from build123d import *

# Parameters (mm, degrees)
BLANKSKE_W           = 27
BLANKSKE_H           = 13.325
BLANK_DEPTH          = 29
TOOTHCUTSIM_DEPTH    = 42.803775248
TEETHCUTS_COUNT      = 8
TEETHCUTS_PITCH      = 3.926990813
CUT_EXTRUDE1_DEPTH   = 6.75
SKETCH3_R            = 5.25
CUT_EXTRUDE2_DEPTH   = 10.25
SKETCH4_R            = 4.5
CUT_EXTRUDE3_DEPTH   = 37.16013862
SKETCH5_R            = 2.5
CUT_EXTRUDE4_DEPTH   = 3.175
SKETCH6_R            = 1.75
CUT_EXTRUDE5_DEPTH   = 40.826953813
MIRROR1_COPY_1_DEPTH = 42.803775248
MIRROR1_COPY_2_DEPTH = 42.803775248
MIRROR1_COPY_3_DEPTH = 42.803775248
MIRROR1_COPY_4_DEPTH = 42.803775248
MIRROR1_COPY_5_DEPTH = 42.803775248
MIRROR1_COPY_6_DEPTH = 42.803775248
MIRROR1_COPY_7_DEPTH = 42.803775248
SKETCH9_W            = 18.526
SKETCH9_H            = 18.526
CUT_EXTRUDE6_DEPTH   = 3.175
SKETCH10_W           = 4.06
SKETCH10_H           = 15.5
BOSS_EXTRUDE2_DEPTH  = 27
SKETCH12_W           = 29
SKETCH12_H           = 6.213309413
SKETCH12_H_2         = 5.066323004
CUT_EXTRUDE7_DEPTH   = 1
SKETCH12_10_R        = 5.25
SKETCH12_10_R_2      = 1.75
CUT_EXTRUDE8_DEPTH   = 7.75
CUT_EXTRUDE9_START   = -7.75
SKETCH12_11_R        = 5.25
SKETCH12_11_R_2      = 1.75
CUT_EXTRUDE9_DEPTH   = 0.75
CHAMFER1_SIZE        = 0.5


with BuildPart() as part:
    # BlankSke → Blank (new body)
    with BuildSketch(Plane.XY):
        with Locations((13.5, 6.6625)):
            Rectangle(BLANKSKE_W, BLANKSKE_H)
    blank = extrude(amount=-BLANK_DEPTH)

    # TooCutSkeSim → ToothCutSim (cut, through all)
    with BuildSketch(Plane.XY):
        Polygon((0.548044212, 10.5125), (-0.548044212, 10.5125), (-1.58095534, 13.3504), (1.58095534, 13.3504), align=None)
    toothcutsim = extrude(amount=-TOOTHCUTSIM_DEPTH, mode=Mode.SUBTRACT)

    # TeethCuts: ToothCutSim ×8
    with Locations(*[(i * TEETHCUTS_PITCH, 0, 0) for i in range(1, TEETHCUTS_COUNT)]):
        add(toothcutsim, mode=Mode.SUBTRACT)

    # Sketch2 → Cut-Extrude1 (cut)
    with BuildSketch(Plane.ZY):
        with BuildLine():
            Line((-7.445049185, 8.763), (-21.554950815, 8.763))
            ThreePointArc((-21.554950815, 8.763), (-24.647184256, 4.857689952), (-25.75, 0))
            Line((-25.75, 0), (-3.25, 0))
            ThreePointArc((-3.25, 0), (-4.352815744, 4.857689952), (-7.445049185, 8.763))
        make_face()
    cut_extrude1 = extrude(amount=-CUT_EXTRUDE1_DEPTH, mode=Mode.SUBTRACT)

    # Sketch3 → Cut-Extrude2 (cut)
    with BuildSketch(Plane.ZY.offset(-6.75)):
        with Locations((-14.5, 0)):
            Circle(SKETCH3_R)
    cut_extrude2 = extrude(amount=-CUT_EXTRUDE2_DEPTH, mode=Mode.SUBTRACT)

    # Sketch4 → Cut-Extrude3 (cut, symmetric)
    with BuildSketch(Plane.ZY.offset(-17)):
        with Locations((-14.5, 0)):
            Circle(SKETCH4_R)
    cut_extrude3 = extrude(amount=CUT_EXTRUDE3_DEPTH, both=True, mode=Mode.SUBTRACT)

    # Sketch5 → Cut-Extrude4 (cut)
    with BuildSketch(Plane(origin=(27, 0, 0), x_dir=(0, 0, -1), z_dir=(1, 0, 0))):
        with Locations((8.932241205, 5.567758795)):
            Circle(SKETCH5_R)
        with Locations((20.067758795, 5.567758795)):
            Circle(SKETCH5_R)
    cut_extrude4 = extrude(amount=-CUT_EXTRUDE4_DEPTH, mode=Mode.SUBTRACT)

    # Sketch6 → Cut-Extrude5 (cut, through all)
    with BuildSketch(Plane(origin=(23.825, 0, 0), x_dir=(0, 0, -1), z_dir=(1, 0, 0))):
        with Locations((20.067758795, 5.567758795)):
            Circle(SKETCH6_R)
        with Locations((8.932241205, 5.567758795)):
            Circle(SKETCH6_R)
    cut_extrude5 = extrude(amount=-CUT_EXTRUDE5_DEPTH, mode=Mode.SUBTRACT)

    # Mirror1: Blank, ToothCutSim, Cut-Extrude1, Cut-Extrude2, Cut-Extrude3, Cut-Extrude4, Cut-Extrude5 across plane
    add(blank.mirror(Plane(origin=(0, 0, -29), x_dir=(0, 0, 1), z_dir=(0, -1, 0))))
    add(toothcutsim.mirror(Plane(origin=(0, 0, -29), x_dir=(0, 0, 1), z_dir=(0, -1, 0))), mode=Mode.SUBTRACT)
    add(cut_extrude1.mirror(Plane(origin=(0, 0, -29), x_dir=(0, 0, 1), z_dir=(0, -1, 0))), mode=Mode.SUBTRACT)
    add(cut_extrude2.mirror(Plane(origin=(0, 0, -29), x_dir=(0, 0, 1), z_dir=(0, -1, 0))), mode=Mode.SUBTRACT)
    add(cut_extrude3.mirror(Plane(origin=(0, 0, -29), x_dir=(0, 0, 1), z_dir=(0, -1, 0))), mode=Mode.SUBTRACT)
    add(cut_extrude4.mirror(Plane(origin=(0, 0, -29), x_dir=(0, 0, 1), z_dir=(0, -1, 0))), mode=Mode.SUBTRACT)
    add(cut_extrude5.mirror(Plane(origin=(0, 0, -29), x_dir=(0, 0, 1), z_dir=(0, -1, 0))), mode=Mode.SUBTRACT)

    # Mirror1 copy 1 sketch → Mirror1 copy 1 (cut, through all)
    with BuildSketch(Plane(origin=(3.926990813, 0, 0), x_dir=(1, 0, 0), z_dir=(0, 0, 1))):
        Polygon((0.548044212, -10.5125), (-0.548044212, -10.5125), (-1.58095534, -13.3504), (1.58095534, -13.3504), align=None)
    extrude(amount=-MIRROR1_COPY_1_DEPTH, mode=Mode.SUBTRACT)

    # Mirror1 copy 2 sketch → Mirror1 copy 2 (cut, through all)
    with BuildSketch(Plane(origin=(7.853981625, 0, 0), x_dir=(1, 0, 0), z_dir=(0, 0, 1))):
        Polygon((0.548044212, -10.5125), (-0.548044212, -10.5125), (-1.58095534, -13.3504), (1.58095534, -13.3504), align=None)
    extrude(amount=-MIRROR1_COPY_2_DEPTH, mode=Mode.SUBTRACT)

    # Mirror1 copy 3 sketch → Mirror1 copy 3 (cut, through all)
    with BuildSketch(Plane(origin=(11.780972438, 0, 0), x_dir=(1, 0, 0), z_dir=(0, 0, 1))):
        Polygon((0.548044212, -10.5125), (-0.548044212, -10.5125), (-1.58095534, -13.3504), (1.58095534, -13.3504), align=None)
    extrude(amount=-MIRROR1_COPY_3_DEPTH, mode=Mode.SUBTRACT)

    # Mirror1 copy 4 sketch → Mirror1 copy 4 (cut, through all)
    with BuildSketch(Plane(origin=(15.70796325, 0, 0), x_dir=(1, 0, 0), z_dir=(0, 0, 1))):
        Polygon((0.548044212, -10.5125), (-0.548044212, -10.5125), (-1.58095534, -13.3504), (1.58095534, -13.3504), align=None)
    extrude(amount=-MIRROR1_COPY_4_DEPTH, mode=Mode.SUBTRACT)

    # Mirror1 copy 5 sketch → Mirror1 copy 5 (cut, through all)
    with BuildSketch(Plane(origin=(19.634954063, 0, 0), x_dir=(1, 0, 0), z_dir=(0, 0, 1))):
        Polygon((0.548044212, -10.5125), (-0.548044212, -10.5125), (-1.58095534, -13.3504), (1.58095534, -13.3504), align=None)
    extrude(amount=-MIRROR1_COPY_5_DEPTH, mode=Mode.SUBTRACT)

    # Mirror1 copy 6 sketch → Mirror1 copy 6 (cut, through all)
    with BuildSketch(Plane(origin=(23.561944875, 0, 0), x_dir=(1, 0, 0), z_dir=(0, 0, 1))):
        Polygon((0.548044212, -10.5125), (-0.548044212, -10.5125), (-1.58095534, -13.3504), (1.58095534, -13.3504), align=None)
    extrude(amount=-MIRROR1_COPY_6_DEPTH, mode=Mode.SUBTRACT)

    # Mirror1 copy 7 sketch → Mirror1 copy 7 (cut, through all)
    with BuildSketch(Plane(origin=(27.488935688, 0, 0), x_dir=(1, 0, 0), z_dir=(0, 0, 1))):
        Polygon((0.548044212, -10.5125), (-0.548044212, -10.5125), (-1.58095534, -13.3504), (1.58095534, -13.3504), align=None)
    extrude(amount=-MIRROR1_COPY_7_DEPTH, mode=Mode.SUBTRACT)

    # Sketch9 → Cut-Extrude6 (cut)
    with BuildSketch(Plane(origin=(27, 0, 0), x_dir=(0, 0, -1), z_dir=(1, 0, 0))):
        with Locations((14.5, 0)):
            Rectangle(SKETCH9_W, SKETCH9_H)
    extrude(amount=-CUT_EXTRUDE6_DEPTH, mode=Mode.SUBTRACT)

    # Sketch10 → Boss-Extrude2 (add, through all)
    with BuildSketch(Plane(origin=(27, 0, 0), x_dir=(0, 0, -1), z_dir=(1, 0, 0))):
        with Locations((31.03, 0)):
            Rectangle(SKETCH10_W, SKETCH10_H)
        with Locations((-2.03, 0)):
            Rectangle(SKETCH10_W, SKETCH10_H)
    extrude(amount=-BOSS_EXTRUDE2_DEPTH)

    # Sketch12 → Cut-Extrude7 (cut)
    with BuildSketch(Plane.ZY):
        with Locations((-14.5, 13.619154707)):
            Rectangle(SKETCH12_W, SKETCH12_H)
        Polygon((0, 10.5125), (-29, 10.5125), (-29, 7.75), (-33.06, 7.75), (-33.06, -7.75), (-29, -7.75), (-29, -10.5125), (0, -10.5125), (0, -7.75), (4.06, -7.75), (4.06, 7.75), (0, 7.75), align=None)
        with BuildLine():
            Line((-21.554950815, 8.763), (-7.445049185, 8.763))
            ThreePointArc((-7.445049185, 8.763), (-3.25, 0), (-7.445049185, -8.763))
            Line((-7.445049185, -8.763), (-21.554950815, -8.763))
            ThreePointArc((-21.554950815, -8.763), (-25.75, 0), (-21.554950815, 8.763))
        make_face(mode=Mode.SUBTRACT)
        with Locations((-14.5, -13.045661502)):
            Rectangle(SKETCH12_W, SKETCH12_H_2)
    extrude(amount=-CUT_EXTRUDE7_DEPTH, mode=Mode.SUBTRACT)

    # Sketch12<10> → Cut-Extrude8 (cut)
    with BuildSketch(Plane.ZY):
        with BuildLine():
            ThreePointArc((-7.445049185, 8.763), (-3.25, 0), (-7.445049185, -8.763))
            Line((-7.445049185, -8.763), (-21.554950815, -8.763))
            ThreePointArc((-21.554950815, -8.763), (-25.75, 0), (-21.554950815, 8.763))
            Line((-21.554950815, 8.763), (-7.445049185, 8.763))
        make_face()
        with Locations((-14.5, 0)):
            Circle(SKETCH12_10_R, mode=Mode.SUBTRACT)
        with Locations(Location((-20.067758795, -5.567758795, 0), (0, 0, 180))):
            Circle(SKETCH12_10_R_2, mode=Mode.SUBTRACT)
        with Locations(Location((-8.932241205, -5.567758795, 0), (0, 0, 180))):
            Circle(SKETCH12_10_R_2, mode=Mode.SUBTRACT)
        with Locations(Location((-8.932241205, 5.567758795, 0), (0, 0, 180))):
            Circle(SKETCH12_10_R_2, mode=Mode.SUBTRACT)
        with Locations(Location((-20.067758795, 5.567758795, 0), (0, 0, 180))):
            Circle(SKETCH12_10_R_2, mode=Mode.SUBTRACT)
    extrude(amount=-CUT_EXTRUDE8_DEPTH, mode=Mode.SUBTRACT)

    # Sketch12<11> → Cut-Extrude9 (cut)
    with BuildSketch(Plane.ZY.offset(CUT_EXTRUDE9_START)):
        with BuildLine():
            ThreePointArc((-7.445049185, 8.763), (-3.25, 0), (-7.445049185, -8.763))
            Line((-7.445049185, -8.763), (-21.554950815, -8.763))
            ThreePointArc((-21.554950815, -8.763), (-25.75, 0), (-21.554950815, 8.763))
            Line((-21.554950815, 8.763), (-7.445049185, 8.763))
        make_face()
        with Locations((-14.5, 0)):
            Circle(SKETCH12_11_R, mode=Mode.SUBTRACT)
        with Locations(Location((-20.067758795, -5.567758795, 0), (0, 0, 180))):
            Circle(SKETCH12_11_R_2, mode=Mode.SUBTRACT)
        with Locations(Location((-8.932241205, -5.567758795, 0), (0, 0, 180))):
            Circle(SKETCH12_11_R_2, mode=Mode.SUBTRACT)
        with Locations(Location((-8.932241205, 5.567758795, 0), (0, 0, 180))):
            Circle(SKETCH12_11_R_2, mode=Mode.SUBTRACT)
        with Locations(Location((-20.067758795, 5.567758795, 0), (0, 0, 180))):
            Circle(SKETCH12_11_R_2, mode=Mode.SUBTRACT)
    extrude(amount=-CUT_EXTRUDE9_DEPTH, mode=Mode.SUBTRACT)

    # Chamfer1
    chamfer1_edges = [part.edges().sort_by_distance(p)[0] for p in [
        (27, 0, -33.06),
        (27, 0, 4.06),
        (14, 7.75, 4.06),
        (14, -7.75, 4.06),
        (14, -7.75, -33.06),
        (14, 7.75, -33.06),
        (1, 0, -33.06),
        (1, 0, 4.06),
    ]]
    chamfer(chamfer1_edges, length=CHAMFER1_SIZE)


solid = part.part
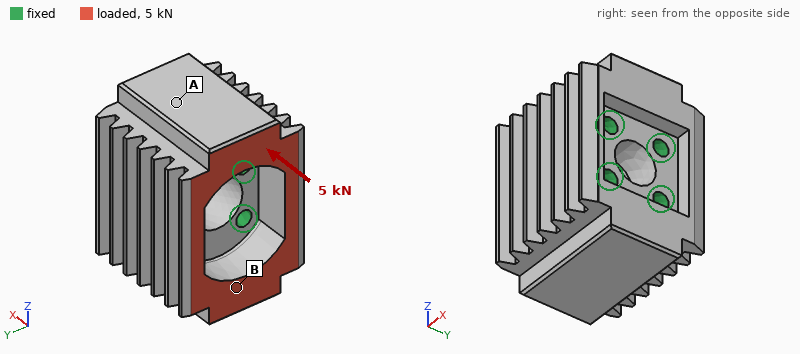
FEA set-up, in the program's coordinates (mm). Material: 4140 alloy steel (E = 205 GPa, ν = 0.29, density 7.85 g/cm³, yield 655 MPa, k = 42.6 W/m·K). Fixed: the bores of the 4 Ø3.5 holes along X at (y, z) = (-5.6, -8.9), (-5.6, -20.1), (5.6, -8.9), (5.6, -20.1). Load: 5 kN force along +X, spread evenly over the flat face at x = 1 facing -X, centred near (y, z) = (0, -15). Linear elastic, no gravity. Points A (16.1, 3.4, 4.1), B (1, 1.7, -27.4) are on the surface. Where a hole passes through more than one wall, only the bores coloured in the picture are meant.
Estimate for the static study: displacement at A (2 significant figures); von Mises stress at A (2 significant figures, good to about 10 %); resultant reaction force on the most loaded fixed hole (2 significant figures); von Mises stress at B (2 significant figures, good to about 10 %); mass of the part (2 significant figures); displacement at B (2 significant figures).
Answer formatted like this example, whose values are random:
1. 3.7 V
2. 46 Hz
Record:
1. 0.95 µm
2. 4.6 MPa
3. 1.3 kN
4. 13 MPa
5. 120 g
6. 1.5 µm
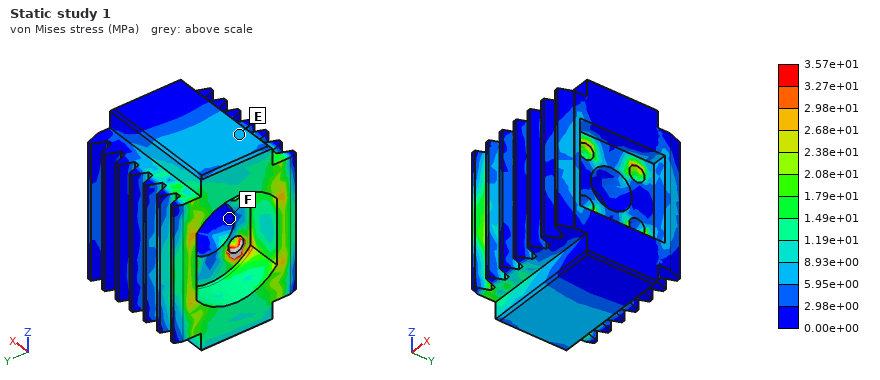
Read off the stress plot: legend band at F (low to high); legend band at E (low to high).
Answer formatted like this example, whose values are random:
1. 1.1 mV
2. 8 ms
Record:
1. 0.00e+00 to 2.98e+00 MPa
2. 5.95e+00 to 8.93e+00 MPa
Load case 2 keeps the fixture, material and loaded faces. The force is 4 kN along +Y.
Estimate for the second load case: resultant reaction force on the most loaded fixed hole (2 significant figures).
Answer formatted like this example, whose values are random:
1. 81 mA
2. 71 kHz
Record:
1. 1.7 kN
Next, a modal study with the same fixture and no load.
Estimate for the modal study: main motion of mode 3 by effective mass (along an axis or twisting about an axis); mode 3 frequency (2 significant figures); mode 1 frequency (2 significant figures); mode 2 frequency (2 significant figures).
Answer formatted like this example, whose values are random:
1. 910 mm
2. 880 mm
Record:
1. along X
2. 34 kHz
3. 32 kHz
4. 32 kHz
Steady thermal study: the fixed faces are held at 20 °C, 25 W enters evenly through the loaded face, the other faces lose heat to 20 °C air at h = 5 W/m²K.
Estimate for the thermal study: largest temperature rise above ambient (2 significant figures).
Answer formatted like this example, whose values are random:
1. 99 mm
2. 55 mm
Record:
1. 20 K
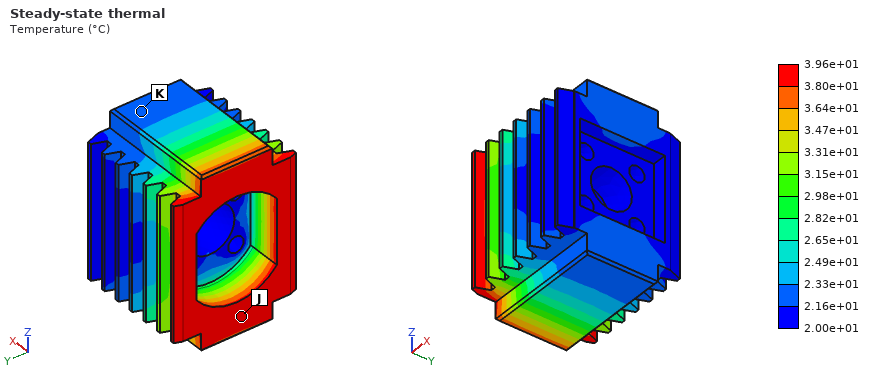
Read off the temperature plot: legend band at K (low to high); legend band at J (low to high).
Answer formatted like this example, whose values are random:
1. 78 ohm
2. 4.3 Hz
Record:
1. 2.16e+01 to 2.33e+01 °C
2. 3.80e+01 to 3.96e+01 °C
